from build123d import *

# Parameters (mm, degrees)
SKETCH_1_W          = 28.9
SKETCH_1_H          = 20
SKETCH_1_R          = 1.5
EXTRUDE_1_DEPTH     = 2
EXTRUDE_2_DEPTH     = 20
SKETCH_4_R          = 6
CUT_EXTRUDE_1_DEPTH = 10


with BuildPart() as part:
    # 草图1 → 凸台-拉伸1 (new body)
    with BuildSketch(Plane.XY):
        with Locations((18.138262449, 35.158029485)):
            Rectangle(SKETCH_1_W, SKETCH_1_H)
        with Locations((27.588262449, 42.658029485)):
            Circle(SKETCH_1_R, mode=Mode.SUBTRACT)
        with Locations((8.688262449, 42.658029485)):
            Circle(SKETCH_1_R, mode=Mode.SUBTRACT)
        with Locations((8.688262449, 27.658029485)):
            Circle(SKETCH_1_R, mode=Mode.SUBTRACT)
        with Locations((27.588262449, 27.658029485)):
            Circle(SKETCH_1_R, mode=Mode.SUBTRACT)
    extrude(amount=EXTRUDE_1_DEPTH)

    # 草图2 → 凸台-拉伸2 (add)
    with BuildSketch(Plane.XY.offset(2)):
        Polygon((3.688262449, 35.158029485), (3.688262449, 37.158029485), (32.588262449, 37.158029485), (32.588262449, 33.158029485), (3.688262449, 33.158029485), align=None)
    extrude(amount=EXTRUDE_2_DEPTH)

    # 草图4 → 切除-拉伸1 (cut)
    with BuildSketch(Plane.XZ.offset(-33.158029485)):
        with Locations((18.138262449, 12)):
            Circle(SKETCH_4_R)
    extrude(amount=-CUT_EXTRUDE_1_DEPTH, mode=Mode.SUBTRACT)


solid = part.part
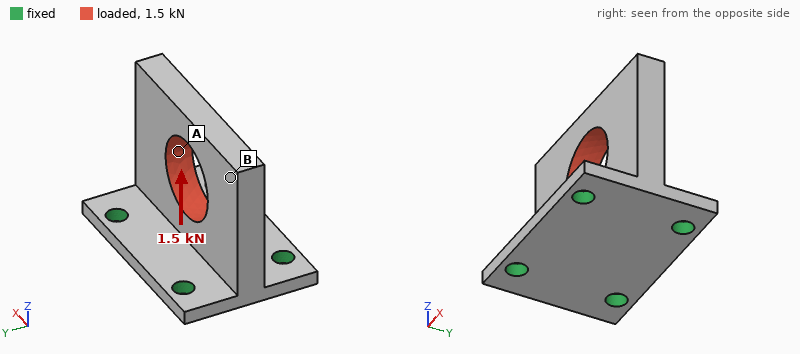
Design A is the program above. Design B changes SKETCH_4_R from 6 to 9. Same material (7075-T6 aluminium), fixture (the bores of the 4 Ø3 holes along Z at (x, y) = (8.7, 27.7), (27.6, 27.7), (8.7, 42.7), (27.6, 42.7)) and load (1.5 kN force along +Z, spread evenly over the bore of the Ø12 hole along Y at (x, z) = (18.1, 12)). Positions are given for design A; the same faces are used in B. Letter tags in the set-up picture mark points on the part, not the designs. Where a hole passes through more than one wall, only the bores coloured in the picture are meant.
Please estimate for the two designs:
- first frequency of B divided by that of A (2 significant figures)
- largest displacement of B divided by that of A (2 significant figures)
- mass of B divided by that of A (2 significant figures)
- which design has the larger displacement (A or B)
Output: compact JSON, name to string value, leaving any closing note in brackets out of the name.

{"first frequency of B divided by that of A": "1.00", "largest displacement of B divided by that of A": "2.3", "mass of B divided by that of A": "0.81", "which design has the larger displacement": "B"}
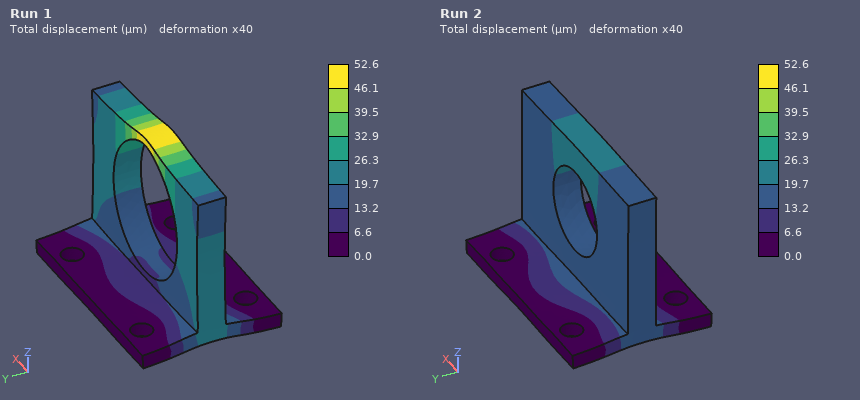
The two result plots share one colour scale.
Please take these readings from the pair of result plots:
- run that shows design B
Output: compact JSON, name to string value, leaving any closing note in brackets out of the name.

{"run that shows design B": "Run 1"}
